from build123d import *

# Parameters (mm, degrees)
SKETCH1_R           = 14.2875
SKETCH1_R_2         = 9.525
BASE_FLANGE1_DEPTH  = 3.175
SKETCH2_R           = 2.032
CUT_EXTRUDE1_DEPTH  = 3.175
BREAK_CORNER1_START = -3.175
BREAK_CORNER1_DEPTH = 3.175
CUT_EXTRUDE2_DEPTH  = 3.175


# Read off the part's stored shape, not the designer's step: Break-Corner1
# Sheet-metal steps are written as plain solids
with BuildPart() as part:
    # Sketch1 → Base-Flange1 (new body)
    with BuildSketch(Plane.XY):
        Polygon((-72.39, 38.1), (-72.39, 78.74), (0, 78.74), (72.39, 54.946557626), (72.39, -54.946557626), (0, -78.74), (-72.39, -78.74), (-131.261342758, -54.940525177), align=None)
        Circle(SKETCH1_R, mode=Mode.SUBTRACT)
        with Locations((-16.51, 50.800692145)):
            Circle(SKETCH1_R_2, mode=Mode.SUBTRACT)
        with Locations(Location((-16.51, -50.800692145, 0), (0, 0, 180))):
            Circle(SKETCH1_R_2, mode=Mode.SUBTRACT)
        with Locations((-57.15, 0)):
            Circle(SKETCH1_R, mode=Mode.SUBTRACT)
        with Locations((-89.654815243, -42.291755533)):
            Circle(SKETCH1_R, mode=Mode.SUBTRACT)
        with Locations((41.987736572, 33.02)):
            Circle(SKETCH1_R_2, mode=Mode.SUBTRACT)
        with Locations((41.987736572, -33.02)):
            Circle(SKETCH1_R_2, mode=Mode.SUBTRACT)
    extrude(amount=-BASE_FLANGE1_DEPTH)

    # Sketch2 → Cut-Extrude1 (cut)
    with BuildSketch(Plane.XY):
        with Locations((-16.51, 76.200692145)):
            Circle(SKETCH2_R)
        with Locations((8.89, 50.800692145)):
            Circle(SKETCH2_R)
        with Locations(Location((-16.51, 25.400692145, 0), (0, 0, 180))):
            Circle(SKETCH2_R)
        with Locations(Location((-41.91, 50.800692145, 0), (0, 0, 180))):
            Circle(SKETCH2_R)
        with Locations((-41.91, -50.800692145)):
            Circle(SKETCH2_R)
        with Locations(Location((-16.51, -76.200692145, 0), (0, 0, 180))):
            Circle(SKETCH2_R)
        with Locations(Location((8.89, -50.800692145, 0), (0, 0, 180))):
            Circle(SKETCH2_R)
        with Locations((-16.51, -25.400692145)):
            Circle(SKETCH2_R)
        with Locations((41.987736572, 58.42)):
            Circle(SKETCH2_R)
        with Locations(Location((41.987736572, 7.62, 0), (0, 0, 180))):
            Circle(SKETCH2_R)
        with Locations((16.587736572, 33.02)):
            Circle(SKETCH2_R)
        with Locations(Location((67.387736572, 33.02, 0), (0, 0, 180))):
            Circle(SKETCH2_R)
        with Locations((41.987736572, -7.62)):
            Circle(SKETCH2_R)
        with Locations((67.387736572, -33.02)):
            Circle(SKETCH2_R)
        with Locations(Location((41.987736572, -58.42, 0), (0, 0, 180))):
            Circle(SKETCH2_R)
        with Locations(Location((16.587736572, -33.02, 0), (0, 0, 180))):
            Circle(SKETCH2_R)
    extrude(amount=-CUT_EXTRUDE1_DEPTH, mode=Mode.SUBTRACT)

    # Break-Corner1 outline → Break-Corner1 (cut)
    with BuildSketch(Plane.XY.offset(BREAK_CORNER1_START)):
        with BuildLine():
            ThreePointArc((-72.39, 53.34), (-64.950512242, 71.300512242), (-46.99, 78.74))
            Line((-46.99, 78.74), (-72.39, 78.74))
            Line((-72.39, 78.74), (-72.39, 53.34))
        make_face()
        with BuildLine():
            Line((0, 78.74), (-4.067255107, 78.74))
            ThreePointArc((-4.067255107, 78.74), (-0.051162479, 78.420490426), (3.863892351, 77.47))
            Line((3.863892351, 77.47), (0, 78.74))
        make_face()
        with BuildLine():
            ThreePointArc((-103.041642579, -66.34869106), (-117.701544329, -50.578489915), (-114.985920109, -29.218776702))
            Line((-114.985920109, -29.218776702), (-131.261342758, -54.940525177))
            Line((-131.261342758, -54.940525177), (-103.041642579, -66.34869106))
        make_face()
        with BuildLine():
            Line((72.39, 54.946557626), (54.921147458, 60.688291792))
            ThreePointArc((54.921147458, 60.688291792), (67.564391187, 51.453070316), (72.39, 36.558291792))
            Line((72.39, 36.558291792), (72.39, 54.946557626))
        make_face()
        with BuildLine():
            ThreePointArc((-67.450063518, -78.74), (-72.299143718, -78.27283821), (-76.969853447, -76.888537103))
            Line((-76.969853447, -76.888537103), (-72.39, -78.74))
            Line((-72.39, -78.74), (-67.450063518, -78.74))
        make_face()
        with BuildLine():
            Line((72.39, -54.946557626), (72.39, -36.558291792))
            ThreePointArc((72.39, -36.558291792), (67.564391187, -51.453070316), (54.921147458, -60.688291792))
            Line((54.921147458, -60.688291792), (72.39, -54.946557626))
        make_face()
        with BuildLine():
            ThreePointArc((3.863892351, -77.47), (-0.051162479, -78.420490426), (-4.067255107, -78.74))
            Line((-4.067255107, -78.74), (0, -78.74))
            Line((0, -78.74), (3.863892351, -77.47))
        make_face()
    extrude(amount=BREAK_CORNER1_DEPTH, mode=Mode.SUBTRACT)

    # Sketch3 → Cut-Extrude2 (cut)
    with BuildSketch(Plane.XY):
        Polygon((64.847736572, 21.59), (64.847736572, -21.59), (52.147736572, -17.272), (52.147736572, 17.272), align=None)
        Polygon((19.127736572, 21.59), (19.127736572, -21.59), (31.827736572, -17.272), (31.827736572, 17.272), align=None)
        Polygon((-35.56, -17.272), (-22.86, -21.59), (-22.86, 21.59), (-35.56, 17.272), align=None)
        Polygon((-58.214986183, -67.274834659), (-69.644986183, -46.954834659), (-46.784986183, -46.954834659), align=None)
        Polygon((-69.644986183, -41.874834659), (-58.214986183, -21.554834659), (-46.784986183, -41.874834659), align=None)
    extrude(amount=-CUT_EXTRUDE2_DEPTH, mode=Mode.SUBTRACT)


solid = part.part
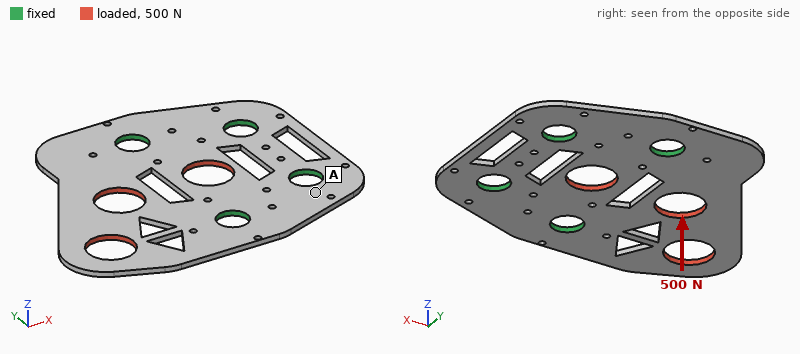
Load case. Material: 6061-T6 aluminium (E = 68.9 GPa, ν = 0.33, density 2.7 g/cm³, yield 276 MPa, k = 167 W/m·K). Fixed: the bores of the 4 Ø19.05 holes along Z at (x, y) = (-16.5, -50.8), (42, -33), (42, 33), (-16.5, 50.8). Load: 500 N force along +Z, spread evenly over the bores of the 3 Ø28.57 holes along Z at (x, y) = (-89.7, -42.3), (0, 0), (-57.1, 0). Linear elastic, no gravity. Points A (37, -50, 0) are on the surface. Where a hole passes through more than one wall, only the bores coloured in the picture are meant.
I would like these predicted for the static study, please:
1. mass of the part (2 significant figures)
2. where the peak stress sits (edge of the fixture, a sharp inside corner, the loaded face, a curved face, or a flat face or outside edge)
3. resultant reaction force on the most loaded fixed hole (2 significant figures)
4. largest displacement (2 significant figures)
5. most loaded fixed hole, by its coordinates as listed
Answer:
160 g
a flat face or outside edge
290 N
2.5 mm
(-16.5, -50.8)
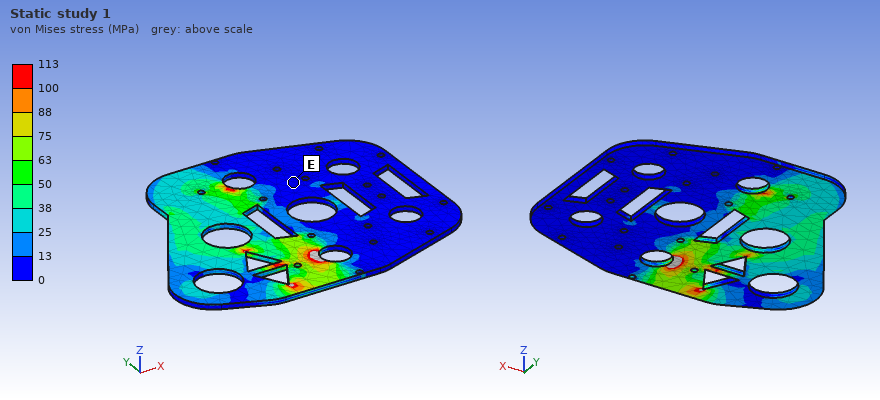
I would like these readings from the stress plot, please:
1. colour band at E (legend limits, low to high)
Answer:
0 to 13 MPa
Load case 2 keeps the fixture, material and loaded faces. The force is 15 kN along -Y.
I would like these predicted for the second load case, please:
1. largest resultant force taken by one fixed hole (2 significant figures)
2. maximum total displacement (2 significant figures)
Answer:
8.4 kN
0.19 mm
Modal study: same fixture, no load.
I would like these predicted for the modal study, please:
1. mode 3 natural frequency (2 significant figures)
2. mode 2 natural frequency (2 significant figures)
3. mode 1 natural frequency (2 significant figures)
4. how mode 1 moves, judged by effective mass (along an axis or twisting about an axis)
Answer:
1500 Hz
880 Hz
370 Hz
along Z
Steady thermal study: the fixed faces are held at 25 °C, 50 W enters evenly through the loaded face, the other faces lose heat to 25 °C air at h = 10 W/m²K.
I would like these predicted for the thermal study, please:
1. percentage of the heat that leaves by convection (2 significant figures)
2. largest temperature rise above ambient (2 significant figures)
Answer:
10 %
52 K
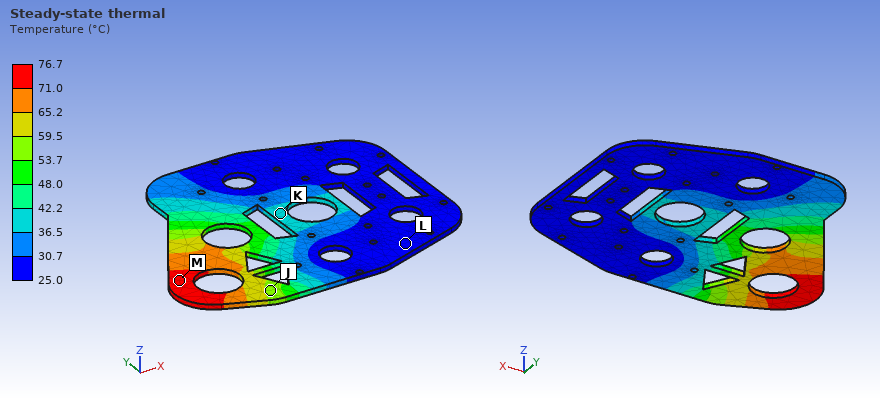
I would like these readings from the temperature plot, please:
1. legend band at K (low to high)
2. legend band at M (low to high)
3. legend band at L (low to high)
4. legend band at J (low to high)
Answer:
36.5 to 42.2 °C
71.0 to 76.7 °C
25.0 to 30.7 °C
53.7 to 59.5 °C
